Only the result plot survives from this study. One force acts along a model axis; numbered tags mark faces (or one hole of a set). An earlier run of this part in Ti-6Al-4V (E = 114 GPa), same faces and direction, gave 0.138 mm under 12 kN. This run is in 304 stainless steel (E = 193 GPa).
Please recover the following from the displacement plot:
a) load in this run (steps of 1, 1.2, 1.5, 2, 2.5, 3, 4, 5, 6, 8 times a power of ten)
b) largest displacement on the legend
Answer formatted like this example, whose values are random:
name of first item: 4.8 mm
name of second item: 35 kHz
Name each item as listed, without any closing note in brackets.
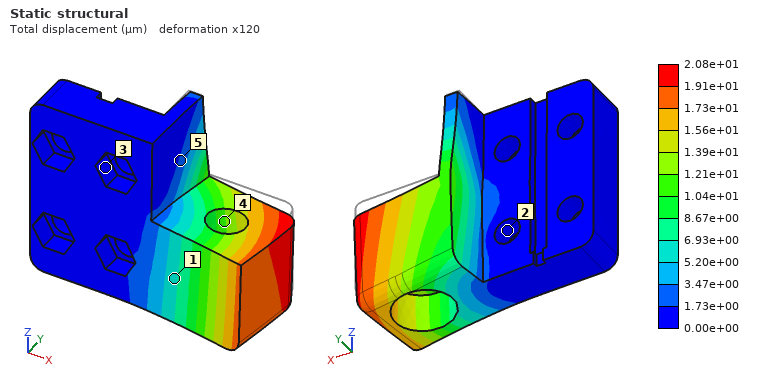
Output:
load in this run: 3 kN
largest displacement on the legend: 2.08e+01 µm
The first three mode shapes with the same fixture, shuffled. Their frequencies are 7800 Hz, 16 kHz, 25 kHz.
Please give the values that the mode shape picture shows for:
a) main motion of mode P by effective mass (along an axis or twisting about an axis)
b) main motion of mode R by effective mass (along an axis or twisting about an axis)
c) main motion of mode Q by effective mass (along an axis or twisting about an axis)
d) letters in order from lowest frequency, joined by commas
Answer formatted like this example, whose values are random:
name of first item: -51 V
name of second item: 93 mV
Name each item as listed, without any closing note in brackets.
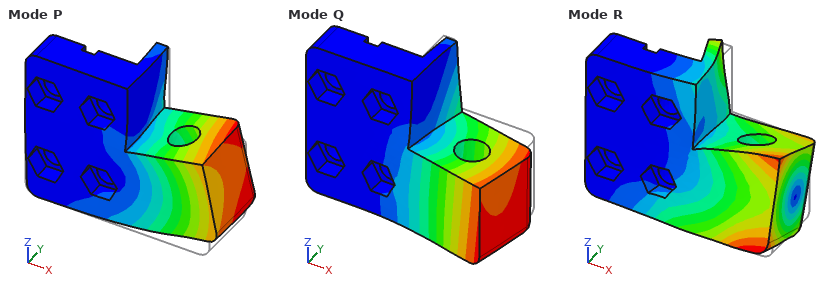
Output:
main motion of mode P by effective mass: along Z
main motion of mode R by effective mass: twisting about X
main motion of mode Q by effective mass: along Y
letters in order from lowest frequency, joined by commas: Q, P, R
